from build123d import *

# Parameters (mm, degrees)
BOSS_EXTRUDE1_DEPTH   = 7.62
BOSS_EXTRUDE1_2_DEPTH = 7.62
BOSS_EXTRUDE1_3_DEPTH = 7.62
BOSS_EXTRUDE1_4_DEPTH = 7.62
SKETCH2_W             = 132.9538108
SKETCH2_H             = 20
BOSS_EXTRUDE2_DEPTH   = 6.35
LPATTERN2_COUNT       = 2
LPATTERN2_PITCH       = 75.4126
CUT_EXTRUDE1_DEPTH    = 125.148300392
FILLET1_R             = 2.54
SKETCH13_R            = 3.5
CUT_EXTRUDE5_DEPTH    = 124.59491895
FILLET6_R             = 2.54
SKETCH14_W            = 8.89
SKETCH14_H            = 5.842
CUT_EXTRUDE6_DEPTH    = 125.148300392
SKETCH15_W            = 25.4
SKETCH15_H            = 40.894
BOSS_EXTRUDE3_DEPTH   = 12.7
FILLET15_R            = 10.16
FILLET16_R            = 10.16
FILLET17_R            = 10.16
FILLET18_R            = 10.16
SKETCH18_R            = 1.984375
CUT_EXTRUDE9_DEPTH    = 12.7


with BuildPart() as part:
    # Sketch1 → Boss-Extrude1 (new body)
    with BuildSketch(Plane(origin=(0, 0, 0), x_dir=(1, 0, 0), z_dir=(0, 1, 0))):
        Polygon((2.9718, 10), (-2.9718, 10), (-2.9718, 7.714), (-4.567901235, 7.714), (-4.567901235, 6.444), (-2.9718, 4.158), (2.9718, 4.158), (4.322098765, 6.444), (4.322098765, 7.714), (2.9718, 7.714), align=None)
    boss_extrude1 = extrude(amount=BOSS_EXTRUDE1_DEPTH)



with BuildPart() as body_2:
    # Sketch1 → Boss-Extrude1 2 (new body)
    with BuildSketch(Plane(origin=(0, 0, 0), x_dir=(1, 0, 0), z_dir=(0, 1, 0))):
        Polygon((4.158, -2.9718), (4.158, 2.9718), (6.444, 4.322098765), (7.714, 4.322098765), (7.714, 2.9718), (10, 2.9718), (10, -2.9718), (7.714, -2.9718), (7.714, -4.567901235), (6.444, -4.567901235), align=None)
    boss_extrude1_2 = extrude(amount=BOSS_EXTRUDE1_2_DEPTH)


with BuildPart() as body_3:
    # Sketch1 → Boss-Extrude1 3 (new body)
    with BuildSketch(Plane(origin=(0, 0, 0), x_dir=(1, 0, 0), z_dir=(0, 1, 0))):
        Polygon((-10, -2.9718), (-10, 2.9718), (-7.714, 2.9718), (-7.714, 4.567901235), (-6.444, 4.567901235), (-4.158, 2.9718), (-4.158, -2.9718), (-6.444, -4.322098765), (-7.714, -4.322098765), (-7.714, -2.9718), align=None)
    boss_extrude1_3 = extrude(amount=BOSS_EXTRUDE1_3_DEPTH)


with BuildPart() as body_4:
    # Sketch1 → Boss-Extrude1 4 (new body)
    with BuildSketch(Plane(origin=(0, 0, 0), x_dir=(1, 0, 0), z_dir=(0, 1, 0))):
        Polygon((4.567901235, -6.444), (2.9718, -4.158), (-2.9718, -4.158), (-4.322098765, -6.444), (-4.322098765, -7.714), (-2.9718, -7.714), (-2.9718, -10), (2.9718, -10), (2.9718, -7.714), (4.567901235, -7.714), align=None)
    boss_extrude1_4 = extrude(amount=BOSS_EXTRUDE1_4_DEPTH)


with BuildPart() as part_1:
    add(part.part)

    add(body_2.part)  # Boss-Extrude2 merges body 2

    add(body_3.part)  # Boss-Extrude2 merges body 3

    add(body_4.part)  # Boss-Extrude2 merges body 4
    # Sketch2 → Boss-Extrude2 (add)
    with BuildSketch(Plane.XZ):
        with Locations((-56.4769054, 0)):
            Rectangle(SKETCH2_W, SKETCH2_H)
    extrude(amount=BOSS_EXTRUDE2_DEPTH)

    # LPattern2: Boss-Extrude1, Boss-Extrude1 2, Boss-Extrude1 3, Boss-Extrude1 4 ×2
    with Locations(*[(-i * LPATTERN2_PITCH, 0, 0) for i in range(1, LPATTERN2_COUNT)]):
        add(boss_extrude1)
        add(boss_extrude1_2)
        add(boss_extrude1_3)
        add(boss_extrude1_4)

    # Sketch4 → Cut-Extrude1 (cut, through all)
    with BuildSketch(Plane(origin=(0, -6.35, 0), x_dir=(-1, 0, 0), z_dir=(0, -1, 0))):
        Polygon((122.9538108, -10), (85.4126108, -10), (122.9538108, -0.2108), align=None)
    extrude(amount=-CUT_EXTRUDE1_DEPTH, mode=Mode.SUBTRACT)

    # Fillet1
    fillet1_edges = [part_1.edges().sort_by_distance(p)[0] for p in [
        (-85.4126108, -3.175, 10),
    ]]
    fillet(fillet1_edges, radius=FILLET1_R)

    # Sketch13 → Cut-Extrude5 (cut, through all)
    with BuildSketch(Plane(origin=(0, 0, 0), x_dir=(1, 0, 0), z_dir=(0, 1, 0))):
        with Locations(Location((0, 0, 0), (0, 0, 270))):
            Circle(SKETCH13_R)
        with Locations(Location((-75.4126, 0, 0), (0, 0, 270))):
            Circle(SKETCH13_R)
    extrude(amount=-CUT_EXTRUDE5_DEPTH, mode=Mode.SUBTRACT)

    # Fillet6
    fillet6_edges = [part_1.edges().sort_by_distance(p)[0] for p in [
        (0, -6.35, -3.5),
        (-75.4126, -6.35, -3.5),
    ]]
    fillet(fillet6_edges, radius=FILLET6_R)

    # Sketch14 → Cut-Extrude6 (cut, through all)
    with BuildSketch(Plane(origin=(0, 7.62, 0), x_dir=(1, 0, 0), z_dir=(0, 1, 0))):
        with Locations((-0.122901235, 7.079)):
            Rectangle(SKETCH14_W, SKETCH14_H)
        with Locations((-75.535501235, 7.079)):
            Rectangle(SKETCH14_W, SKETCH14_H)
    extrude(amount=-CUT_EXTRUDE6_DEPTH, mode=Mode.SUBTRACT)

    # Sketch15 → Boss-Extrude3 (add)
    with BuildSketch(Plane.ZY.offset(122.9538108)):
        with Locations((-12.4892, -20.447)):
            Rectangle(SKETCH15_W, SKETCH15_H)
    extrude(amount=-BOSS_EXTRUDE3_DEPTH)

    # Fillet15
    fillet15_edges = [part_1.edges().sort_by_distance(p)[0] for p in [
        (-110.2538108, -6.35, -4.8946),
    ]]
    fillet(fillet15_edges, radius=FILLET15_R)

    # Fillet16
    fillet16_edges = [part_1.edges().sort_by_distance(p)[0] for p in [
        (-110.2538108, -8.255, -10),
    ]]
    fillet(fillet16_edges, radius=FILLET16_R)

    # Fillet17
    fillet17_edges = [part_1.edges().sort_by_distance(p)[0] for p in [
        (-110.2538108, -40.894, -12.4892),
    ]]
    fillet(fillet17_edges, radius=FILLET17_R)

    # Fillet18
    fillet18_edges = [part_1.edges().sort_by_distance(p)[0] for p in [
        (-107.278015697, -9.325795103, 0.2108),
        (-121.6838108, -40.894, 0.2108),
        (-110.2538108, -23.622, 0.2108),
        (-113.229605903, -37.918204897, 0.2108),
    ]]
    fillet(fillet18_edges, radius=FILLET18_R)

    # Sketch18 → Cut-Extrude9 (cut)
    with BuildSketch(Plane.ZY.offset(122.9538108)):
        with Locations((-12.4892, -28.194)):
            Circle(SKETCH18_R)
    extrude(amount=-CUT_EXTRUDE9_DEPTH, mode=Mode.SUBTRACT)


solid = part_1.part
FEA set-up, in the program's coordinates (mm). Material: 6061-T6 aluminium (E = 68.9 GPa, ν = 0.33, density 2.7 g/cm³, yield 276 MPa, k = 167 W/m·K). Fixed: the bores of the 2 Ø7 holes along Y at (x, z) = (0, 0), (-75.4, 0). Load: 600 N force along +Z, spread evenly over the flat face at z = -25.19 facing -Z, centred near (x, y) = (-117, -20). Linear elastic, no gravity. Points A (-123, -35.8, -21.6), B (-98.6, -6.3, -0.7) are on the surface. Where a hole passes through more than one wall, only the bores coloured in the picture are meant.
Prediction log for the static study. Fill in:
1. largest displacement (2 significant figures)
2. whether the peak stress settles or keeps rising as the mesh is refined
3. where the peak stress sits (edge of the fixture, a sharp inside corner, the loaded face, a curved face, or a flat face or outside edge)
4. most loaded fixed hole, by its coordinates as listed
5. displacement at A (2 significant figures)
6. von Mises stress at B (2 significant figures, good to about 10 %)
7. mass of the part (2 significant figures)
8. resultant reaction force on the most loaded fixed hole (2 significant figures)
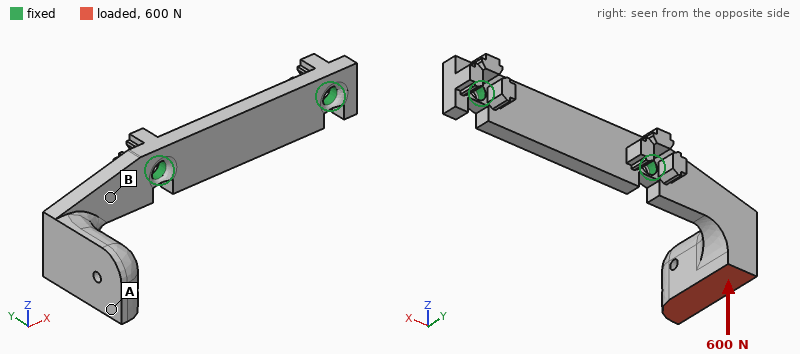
0.68 mm
keeps rising
edge of the fixture
(-75.4, 0)
0.61 mm
100 MPa
75 g
710 N
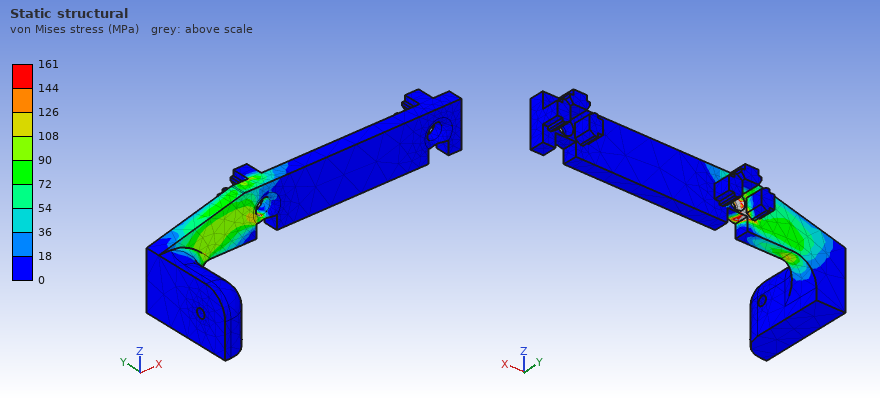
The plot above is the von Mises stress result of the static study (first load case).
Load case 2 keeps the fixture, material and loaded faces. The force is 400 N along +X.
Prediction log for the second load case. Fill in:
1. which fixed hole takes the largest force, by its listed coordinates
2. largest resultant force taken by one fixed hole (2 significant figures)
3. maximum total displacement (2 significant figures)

(-75.4, 0)
440 N
0.55 mm
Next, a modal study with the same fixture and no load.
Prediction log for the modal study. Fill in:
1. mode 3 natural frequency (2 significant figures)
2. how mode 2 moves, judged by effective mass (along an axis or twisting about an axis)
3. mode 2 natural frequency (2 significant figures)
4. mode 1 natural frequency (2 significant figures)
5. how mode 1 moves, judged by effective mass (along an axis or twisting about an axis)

2700 Hz
along Z
1100 Hz
660 Hz
along Y
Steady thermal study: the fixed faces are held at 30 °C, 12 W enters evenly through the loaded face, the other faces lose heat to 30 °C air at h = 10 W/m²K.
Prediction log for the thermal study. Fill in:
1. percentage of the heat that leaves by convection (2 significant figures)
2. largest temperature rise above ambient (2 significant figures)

7.9 %
29 K
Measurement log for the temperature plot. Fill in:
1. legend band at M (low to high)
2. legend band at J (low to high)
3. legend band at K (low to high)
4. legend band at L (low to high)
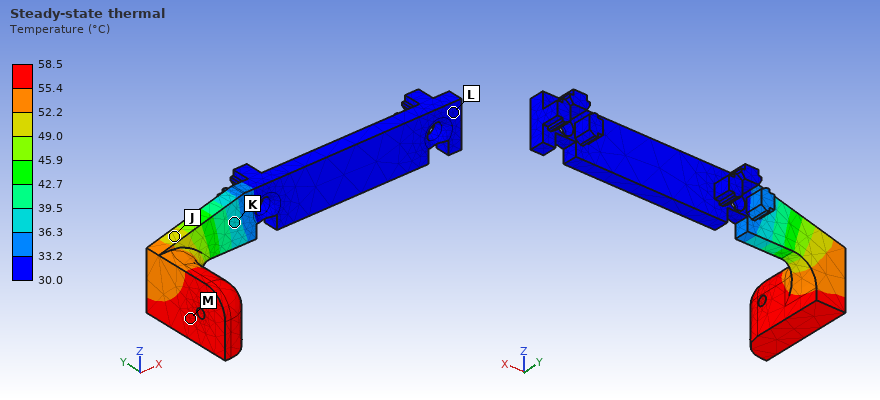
55.4 to 58.5 °C
49.0 to 52.2 °C
36.3 to 39.5 °C
30.0 to 33.2 °C
